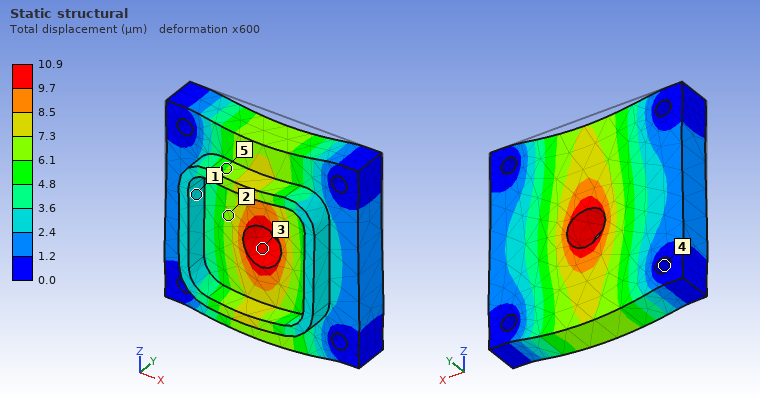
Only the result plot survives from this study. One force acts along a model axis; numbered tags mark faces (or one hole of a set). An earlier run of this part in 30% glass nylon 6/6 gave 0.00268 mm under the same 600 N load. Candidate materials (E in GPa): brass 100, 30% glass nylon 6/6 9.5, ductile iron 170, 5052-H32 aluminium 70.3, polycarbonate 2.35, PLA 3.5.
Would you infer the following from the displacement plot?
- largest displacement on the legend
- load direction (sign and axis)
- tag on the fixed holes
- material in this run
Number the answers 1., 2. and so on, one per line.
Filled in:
1. 10.9 µm
2. -Z
3. 4
4. polycarbonate
